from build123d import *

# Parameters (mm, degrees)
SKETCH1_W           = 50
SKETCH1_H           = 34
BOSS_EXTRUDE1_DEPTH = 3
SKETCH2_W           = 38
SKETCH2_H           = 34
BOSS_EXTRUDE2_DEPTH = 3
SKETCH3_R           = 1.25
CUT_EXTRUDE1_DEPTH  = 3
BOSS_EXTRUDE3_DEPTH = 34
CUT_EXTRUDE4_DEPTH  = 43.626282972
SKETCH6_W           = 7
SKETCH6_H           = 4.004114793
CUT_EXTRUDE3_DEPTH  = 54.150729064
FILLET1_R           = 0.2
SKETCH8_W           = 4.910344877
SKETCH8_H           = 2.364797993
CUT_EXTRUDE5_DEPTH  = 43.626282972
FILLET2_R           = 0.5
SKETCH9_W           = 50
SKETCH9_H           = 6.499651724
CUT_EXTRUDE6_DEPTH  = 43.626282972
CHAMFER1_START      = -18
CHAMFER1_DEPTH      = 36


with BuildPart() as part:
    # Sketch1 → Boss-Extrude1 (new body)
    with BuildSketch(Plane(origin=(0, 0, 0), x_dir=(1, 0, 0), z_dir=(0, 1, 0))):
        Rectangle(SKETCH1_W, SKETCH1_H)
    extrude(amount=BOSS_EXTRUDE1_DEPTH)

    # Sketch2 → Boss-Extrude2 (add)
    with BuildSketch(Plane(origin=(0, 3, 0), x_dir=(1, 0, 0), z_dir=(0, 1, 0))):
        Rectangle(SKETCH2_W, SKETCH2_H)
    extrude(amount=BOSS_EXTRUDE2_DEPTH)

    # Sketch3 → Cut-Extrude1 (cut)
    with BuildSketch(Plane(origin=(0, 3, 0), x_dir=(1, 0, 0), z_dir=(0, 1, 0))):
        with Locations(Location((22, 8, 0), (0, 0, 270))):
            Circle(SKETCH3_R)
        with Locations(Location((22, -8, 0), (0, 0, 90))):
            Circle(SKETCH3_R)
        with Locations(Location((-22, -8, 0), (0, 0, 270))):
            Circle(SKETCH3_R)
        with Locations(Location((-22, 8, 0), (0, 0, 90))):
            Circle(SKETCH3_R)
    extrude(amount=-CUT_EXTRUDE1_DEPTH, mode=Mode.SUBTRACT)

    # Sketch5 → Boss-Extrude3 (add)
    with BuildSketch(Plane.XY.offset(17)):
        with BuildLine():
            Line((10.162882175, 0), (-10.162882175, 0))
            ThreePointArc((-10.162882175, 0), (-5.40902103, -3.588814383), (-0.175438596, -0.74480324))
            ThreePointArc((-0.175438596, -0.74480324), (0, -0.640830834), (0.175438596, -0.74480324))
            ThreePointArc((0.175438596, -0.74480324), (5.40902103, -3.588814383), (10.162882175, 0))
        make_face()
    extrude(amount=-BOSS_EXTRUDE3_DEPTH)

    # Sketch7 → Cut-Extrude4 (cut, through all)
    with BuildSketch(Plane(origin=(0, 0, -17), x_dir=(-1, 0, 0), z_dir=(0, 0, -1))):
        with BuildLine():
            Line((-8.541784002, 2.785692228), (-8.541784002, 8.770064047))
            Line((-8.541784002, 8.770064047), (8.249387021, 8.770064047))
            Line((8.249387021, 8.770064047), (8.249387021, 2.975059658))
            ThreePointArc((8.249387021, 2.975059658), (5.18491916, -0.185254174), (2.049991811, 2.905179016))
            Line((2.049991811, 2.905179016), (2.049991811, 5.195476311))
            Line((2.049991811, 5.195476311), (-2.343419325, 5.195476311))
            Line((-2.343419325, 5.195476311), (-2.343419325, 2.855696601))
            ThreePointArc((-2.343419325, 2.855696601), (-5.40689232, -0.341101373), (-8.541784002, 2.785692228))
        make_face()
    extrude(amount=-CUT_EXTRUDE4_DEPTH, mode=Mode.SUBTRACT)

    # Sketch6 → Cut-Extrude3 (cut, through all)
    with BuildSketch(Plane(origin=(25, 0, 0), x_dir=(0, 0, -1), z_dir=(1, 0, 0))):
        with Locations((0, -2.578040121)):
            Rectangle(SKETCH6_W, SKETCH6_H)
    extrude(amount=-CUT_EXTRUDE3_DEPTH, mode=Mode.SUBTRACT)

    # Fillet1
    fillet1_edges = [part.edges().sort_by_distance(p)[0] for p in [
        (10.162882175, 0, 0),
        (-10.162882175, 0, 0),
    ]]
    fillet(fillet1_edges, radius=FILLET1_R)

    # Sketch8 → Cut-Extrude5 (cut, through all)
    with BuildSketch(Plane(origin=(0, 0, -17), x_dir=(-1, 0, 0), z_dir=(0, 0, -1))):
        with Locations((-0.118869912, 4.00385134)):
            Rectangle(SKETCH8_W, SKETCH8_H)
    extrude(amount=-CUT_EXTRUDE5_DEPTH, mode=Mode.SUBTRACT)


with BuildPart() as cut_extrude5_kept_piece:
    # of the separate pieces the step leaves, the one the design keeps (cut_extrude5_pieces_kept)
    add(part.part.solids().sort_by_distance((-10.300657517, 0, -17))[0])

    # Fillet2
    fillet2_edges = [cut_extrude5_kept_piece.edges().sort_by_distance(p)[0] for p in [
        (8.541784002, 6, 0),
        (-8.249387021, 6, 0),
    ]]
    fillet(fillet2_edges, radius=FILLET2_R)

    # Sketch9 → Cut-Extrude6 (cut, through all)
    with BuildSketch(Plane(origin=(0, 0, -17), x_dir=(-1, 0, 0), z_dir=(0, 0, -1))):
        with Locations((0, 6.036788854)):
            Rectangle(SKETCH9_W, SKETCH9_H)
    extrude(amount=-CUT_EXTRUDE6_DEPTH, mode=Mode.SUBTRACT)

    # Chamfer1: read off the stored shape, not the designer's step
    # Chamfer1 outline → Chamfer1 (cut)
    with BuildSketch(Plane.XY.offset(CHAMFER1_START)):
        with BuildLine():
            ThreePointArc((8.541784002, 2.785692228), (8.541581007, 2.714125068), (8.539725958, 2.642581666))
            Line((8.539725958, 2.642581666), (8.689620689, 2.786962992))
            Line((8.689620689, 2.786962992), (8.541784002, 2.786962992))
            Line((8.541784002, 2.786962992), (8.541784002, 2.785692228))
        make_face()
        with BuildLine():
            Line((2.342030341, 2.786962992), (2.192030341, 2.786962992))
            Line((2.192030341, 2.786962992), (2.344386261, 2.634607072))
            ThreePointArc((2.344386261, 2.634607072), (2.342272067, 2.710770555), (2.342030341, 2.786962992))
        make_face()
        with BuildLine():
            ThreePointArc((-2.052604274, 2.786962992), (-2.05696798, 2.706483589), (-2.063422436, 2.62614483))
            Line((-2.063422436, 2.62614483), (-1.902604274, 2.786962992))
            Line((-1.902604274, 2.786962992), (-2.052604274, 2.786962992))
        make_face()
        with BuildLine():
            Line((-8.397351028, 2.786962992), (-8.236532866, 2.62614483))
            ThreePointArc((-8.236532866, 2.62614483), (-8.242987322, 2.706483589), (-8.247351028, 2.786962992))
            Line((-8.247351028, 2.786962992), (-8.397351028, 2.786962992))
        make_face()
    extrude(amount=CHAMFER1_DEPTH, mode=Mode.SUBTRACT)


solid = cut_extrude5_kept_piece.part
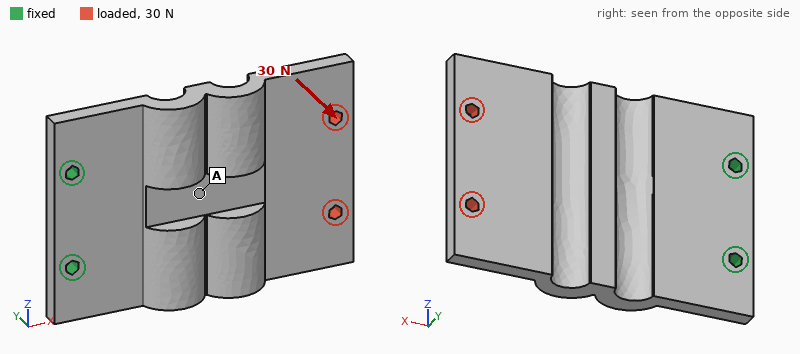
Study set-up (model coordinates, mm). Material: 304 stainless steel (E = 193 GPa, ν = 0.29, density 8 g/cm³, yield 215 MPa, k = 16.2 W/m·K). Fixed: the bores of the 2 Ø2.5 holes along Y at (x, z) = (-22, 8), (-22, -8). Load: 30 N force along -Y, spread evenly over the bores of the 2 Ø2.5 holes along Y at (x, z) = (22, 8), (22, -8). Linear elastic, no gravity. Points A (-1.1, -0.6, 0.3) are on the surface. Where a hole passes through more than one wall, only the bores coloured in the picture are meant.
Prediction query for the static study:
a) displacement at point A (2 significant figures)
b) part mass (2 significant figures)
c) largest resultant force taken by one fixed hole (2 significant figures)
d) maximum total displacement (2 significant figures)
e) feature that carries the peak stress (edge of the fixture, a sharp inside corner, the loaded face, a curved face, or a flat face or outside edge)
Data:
23 µm
42 g
15 N
84 µm
a flat face or outside edge
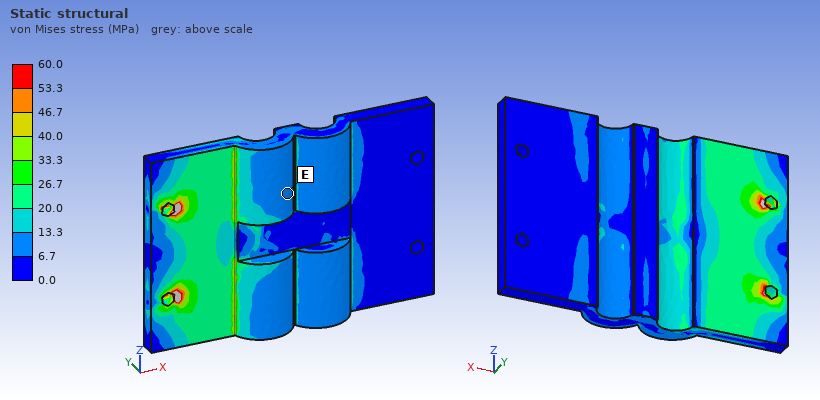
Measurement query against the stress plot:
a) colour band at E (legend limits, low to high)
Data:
6.7 to 13.3 MPa
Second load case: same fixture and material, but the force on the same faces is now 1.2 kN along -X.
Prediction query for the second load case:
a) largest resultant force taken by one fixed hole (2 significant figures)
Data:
600 N
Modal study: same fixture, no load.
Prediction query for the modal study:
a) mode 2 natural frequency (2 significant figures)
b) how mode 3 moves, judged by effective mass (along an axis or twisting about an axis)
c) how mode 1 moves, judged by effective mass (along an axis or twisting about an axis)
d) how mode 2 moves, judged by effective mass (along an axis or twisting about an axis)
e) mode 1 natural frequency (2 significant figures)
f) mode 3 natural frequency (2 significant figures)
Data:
3000 Hz
along Y
along Y
twisting about X
950 Hz
5300 Hz
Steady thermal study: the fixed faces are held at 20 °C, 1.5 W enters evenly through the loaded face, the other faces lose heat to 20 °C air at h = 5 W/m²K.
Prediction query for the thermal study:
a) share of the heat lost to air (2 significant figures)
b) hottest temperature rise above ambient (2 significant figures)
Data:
28 %
43 K
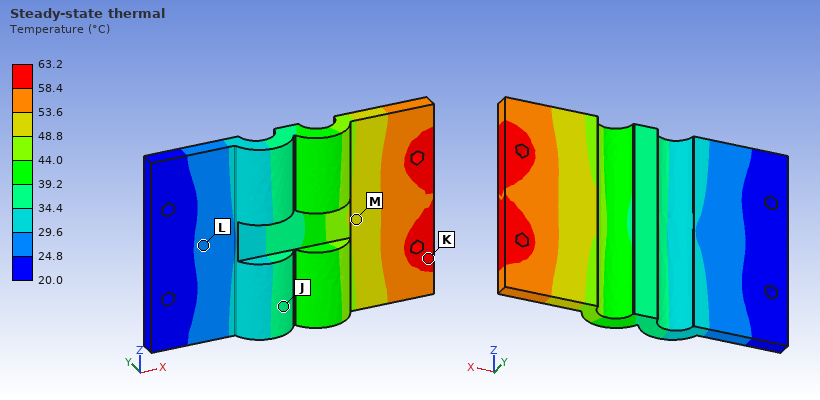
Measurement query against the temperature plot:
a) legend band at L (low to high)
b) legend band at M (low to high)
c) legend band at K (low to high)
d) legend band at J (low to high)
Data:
24.8 to 29.6 °C
48.8 to 53.6 °C
58.4 to 63.2 °C
34.4 to 39.2 °C
